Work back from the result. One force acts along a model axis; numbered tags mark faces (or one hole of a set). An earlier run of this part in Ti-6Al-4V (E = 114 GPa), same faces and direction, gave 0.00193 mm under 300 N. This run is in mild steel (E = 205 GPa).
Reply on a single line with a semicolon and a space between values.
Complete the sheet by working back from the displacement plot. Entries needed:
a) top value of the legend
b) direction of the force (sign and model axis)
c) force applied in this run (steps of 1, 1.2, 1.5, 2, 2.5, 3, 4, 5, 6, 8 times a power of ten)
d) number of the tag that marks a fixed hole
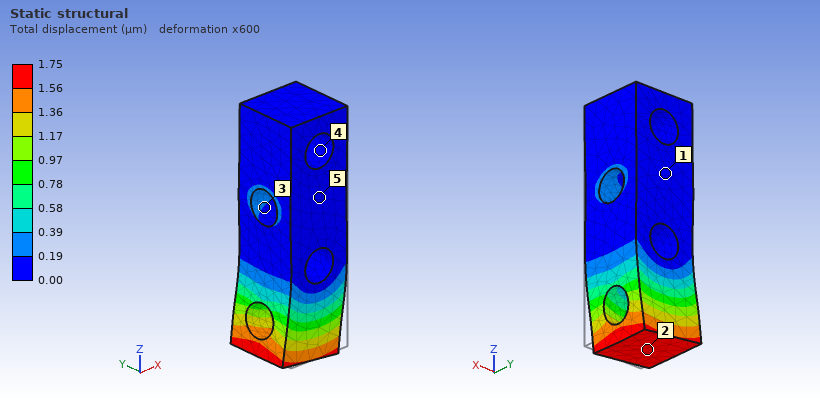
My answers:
1.75 µm; -X; 500 N; 4
